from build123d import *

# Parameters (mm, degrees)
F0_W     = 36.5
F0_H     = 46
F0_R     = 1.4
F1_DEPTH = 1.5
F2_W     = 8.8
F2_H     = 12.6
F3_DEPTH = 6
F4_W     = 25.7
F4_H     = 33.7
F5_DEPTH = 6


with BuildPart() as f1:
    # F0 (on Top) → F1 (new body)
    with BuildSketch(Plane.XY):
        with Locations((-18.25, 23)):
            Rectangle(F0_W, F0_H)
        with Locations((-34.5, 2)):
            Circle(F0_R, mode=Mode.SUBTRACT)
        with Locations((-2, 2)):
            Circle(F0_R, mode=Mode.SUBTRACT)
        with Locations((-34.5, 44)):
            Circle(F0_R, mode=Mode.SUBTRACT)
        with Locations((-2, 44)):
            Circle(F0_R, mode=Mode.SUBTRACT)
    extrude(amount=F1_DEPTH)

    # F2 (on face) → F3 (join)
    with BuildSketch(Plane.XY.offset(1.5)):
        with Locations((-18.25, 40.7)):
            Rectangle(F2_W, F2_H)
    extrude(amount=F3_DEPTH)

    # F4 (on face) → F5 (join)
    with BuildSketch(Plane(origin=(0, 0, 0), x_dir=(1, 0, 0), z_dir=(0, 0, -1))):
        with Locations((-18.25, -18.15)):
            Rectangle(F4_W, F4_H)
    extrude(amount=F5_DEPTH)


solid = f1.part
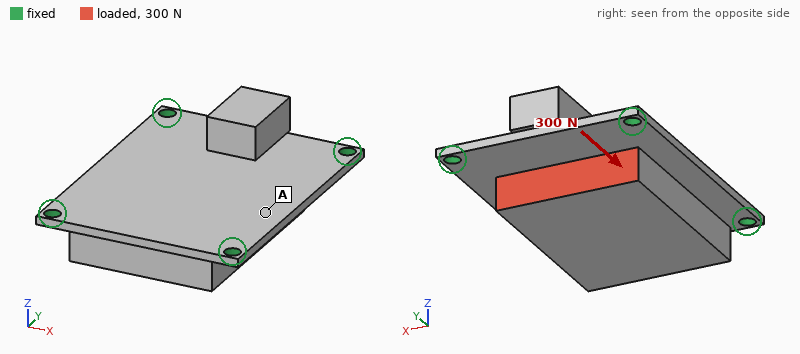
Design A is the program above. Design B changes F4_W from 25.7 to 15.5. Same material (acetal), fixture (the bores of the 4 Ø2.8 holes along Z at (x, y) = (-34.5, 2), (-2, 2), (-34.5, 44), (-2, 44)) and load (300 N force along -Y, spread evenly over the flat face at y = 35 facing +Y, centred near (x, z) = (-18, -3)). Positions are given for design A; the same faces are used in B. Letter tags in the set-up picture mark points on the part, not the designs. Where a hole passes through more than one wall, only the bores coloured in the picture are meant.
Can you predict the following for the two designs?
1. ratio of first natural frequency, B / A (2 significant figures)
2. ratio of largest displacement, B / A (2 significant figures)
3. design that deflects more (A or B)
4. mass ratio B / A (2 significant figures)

0.87
1.6
B
0.75
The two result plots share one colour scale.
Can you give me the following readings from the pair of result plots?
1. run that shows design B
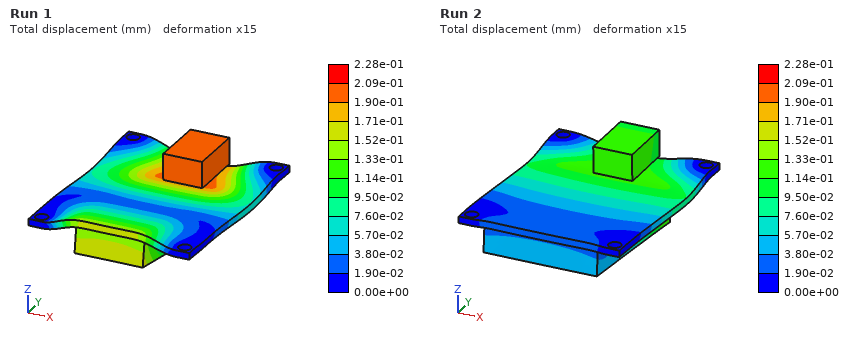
Run 1
